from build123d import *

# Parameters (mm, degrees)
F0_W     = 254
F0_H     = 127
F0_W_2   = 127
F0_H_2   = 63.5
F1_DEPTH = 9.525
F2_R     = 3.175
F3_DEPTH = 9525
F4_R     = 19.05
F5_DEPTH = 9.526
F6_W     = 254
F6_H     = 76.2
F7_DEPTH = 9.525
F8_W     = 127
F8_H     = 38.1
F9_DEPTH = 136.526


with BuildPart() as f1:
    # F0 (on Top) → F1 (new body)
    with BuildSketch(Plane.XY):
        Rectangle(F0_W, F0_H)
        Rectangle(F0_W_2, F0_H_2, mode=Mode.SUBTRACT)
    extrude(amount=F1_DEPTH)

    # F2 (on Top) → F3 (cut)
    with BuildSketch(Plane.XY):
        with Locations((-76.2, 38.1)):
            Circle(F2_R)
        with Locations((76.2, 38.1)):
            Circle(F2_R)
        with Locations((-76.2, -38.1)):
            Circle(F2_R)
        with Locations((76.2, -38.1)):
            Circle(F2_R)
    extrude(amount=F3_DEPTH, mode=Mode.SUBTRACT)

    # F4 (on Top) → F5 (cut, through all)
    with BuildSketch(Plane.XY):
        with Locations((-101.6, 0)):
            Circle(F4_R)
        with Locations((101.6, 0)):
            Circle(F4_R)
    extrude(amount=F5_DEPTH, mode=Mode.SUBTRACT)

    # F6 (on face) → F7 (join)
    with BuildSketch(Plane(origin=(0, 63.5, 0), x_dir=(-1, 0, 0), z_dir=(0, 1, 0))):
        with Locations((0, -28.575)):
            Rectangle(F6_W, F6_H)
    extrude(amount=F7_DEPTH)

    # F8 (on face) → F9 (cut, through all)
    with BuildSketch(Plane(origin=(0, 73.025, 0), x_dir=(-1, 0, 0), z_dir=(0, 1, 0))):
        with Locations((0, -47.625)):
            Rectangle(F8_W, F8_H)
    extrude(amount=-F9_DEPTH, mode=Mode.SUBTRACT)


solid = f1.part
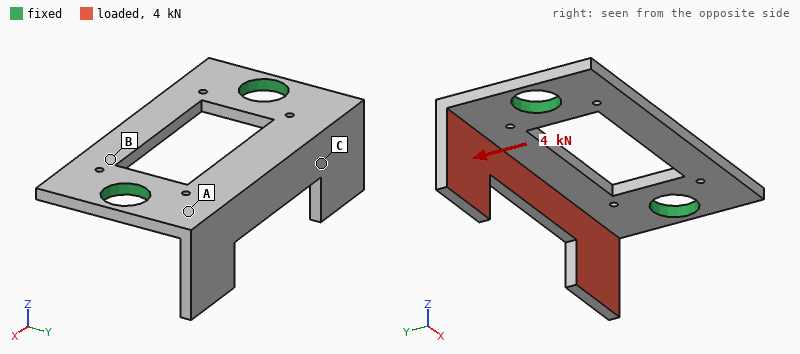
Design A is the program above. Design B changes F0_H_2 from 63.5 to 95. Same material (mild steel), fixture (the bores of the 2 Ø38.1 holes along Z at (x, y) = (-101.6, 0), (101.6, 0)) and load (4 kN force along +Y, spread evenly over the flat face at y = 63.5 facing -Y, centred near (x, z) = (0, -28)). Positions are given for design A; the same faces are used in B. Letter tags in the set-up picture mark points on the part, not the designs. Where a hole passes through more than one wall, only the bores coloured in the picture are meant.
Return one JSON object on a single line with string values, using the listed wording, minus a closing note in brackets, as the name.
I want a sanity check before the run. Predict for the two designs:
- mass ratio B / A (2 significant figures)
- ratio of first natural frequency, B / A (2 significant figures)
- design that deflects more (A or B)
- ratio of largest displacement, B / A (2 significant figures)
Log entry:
{"mass ratio B / A": "0.89", "ratio of first natural frequency, B / A": "0.97", "design that deflects more": "B", "ratio of largest displacement, B / A": "1.1"}
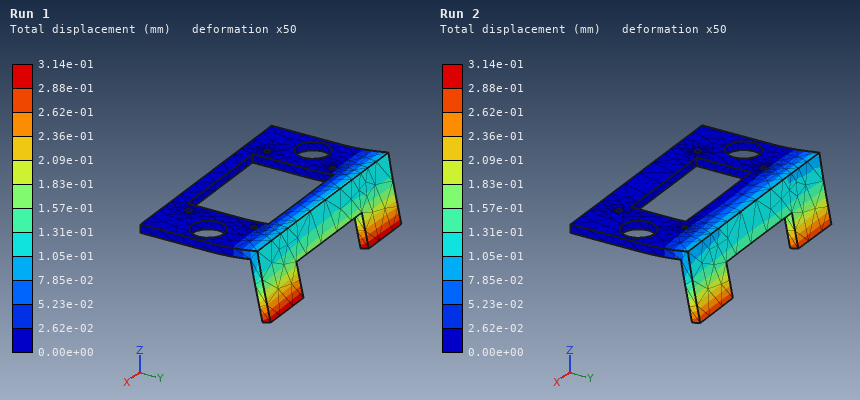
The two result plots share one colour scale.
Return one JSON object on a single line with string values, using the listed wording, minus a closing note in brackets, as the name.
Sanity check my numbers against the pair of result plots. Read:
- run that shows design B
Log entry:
{"run that shows design B": "Run 1"}
